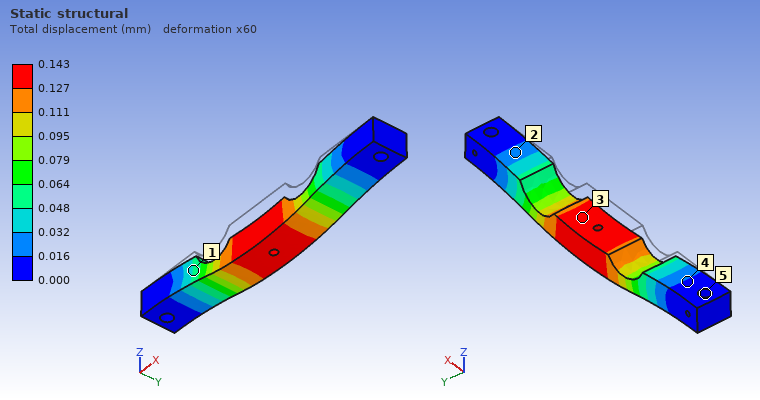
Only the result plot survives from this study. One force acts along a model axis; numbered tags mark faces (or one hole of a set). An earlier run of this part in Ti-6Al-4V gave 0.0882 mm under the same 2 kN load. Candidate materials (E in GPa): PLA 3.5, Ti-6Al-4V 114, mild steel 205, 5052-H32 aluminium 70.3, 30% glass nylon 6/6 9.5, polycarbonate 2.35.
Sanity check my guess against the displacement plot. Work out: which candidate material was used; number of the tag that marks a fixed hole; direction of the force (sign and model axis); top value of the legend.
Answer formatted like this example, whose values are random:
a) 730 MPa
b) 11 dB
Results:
a) 5052-H32 aluminium
b) 5
c) -Z
d) 0.143 mm
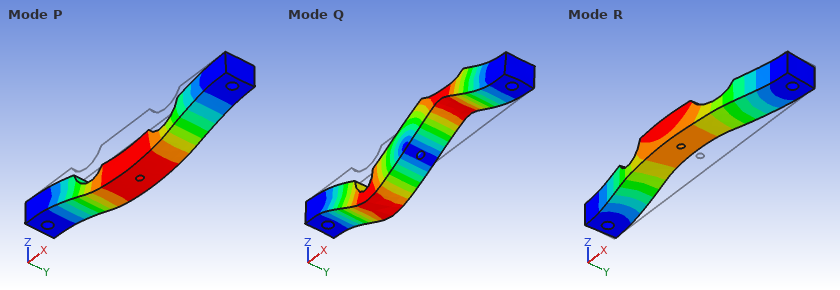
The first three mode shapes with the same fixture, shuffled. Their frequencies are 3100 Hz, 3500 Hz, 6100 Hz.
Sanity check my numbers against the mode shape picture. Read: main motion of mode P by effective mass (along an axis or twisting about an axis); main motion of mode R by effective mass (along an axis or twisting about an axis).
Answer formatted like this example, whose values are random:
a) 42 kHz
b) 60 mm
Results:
a) along Z
b) along Y
